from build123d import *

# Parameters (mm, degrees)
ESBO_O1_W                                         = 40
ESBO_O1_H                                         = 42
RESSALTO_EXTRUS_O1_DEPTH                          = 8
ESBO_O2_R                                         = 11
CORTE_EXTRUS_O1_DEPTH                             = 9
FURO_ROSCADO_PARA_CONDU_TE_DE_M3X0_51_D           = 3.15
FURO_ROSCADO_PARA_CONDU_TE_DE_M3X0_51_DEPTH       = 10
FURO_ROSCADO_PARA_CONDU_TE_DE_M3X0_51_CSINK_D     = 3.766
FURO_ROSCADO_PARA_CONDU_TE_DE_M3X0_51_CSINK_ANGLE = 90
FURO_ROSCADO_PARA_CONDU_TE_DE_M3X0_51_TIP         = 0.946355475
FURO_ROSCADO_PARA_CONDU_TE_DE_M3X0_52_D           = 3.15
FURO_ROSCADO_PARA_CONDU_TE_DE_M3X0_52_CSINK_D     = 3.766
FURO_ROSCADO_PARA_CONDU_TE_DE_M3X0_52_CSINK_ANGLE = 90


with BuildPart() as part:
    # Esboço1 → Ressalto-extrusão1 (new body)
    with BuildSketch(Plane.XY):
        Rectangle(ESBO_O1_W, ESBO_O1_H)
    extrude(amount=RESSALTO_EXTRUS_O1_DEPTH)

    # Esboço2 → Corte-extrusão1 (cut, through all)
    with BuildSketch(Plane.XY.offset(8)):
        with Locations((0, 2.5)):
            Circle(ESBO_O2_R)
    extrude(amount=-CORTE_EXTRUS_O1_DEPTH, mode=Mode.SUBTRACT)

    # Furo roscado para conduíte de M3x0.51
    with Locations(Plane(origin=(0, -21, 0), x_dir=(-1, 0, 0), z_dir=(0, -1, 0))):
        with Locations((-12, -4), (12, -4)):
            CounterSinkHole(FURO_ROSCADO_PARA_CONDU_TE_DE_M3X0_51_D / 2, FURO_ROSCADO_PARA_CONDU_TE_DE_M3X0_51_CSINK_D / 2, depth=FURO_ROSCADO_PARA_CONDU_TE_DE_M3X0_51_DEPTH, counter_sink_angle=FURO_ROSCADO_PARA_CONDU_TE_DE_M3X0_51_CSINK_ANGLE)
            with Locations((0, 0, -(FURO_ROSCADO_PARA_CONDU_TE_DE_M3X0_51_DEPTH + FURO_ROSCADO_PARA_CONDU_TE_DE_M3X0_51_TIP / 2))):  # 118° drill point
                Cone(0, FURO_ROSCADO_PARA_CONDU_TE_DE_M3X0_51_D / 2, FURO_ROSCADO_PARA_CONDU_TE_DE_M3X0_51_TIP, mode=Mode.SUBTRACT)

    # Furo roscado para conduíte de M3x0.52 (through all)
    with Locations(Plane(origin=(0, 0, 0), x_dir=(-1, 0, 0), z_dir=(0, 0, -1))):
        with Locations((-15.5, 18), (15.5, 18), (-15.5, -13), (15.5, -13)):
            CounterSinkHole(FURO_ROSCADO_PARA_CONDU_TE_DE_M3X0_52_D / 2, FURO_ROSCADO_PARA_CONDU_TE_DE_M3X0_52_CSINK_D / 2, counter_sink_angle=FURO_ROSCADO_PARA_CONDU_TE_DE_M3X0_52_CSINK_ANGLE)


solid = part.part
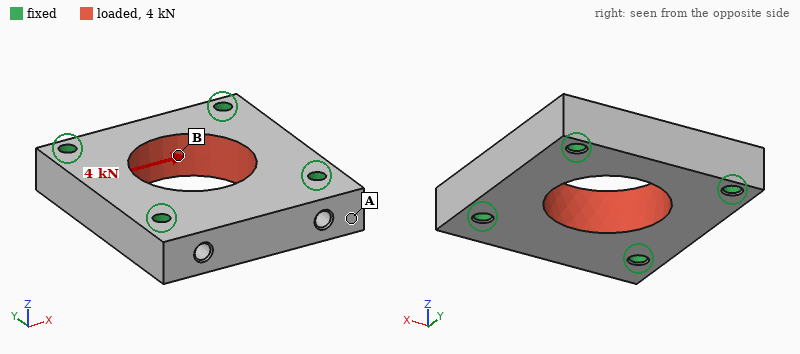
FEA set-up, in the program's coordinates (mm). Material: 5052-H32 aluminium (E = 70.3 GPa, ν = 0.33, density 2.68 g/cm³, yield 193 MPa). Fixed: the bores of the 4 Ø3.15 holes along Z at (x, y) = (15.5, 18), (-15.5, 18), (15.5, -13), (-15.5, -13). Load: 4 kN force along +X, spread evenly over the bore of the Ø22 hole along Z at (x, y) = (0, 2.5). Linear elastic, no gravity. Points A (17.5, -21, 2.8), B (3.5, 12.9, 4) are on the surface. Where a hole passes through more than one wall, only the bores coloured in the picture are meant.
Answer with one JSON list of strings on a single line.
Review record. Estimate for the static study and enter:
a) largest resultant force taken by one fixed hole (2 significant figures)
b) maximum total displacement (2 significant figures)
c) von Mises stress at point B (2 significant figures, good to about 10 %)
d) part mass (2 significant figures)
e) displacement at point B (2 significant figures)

["1.1 kN", "5.4 µm", "16 MPa", "27 g", "2.4 µm"]
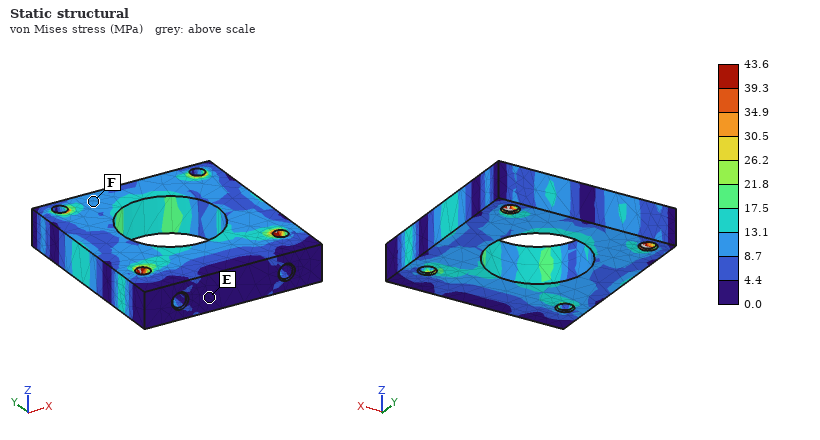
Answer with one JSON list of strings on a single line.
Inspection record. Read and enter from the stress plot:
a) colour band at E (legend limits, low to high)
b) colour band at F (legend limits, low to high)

["0.0 to 4.4 MPa", "8.7 to 13.1 MPa"]
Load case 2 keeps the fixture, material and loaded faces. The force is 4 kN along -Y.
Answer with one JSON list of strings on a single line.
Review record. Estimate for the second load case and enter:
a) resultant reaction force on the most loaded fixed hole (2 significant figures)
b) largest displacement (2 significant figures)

["1.0 kN", "6.3 µm"]
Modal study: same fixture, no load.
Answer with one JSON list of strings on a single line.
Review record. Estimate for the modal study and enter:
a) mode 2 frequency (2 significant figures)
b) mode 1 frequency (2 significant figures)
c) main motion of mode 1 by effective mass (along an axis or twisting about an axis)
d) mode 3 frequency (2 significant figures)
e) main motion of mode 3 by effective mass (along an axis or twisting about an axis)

["27 kHz", "26 kHz", "along Z", "30 kHz", "along Z"]
